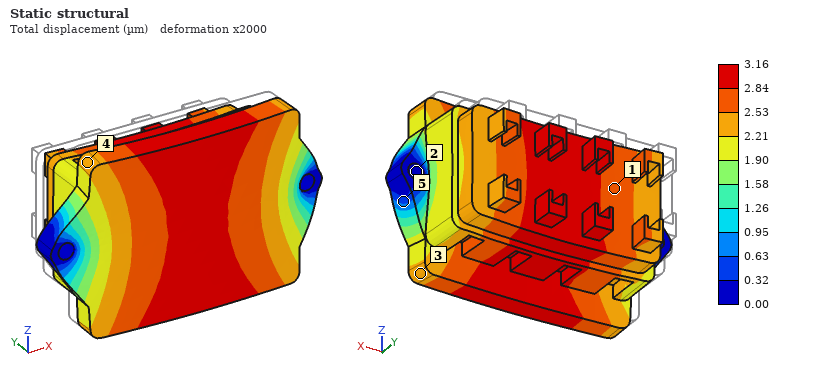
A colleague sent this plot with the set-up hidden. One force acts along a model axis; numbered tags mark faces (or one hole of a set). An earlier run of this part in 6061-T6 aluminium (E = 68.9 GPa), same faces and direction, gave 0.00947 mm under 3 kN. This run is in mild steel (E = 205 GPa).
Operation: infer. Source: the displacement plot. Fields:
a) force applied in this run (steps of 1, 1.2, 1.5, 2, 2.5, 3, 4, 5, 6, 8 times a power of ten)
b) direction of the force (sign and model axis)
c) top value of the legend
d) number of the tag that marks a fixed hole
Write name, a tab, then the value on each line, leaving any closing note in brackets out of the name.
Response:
force applied in this run	3 kN
direction of the force	-Y
top value of the legend	3.16 µm
number of the tag that marks a fixed hole	2
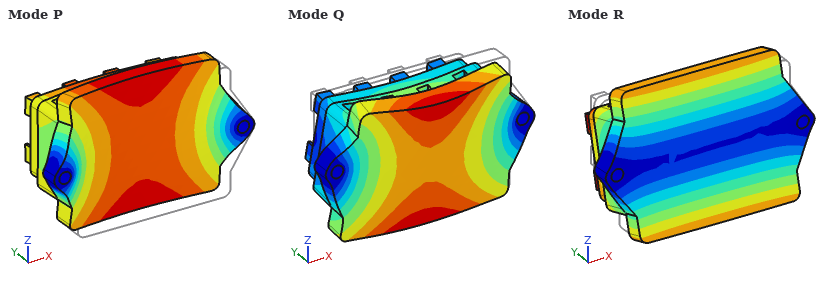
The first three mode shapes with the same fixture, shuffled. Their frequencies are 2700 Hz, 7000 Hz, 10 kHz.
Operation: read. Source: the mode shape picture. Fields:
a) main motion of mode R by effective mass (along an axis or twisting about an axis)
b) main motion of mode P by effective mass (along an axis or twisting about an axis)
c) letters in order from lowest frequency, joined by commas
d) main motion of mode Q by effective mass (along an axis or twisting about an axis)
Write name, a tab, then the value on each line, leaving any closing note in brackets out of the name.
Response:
main motion of mode R by effective mass	along Z
main motion of mode P by effective mass	along Y
letters in order from lowest frequency, joined by commas	R, P, Q
main motion of mode Q by effective mass	along Z
